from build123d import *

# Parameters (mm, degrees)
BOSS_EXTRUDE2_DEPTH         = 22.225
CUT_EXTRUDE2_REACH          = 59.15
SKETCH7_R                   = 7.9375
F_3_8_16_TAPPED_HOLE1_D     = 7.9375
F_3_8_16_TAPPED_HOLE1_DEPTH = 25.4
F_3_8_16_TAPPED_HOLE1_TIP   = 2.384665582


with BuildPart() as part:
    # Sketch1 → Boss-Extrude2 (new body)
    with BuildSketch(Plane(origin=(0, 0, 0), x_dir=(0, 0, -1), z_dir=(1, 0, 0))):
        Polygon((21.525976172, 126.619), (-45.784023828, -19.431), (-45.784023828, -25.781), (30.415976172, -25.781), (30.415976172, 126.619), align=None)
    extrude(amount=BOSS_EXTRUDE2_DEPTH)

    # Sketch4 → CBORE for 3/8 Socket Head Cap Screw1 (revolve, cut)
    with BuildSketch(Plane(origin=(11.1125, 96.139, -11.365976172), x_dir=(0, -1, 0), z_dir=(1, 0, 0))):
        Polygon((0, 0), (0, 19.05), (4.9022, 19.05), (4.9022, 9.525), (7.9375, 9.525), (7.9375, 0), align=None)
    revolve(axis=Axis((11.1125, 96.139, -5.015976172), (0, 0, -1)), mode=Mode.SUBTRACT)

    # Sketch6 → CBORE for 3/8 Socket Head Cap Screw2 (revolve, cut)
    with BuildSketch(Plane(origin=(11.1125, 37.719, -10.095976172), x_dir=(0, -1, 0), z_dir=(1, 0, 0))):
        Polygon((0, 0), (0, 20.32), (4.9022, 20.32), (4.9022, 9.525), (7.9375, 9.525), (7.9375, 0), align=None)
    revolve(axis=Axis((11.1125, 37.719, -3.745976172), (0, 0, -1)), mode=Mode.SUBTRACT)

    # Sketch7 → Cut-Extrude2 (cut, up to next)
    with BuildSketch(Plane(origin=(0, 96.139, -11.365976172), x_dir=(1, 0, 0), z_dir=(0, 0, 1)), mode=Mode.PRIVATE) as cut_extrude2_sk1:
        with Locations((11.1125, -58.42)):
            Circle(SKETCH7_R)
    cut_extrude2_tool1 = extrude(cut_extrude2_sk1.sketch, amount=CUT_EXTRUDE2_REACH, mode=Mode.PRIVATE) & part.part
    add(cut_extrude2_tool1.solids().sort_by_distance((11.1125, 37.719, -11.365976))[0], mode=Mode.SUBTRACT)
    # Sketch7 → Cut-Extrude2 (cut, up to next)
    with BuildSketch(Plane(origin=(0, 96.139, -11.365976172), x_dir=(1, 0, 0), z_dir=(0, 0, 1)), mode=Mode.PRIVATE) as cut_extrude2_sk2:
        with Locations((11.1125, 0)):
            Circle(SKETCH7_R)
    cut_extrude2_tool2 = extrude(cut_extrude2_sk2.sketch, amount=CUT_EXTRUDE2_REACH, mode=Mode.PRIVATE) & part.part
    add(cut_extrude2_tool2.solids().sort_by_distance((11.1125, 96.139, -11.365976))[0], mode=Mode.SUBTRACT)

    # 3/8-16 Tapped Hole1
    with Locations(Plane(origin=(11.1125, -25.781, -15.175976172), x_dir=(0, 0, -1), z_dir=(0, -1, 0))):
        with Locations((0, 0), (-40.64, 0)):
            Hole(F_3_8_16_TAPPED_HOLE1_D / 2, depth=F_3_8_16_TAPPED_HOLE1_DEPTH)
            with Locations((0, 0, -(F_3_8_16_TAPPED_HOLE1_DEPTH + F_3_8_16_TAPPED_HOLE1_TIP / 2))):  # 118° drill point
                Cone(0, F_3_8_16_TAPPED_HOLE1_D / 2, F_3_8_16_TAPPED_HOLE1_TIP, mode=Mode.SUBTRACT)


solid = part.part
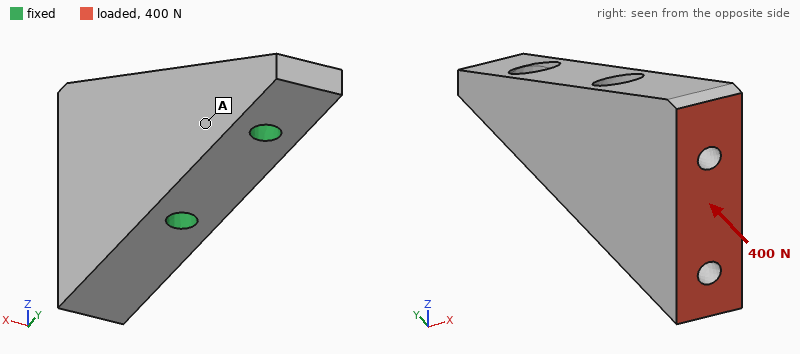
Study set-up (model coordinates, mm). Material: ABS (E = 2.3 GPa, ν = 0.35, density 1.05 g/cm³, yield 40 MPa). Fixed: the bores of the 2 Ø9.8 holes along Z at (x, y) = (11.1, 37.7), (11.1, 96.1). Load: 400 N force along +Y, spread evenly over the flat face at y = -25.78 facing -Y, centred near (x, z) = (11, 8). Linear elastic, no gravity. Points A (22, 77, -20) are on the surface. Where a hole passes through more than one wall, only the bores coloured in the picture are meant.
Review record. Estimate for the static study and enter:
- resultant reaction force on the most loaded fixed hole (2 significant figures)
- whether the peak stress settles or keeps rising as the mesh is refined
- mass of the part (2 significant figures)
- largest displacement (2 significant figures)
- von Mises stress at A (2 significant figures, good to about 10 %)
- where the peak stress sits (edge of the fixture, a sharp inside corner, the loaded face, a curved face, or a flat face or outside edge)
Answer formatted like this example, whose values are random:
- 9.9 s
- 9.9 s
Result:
- 300 N
- keeps rising
- 140 g
- 0.15 mm
- 0.57 MPa
- edge of the fixture
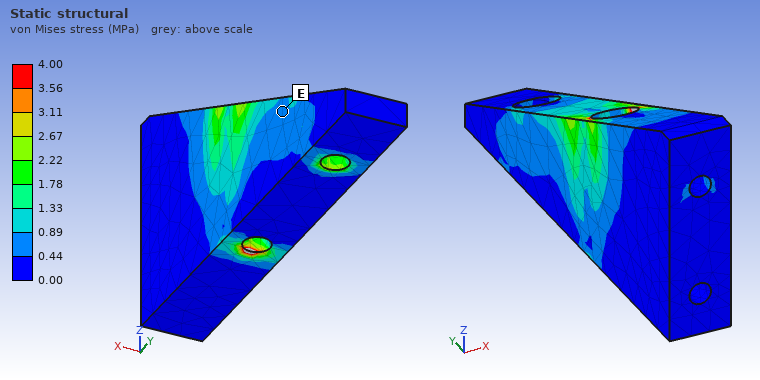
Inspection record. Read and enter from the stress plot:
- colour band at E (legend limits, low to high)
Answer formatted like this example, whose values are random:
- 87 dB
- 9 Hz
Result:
- 0.44 to 0.89 MPa
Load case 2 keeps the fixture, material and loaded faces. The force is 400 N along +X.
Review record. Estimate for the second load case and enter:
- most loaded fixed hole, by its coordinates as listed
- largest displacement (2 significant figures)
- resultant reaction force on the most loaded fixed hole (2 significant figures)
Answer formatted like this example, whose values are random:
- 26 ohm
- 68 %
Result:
- (11.1, 37.7)
- 1.2 mm
- 660 N
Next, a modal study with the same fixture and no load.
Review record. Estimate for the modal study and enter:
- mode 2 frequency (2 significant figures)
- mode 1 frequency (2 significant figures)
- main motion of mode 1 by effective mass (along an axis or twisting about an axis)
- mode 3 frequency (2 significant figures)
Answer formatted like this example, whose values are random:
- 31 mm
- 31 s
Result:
- 900 Hz
- 530 Hz
- along X
- 1200 Hz
